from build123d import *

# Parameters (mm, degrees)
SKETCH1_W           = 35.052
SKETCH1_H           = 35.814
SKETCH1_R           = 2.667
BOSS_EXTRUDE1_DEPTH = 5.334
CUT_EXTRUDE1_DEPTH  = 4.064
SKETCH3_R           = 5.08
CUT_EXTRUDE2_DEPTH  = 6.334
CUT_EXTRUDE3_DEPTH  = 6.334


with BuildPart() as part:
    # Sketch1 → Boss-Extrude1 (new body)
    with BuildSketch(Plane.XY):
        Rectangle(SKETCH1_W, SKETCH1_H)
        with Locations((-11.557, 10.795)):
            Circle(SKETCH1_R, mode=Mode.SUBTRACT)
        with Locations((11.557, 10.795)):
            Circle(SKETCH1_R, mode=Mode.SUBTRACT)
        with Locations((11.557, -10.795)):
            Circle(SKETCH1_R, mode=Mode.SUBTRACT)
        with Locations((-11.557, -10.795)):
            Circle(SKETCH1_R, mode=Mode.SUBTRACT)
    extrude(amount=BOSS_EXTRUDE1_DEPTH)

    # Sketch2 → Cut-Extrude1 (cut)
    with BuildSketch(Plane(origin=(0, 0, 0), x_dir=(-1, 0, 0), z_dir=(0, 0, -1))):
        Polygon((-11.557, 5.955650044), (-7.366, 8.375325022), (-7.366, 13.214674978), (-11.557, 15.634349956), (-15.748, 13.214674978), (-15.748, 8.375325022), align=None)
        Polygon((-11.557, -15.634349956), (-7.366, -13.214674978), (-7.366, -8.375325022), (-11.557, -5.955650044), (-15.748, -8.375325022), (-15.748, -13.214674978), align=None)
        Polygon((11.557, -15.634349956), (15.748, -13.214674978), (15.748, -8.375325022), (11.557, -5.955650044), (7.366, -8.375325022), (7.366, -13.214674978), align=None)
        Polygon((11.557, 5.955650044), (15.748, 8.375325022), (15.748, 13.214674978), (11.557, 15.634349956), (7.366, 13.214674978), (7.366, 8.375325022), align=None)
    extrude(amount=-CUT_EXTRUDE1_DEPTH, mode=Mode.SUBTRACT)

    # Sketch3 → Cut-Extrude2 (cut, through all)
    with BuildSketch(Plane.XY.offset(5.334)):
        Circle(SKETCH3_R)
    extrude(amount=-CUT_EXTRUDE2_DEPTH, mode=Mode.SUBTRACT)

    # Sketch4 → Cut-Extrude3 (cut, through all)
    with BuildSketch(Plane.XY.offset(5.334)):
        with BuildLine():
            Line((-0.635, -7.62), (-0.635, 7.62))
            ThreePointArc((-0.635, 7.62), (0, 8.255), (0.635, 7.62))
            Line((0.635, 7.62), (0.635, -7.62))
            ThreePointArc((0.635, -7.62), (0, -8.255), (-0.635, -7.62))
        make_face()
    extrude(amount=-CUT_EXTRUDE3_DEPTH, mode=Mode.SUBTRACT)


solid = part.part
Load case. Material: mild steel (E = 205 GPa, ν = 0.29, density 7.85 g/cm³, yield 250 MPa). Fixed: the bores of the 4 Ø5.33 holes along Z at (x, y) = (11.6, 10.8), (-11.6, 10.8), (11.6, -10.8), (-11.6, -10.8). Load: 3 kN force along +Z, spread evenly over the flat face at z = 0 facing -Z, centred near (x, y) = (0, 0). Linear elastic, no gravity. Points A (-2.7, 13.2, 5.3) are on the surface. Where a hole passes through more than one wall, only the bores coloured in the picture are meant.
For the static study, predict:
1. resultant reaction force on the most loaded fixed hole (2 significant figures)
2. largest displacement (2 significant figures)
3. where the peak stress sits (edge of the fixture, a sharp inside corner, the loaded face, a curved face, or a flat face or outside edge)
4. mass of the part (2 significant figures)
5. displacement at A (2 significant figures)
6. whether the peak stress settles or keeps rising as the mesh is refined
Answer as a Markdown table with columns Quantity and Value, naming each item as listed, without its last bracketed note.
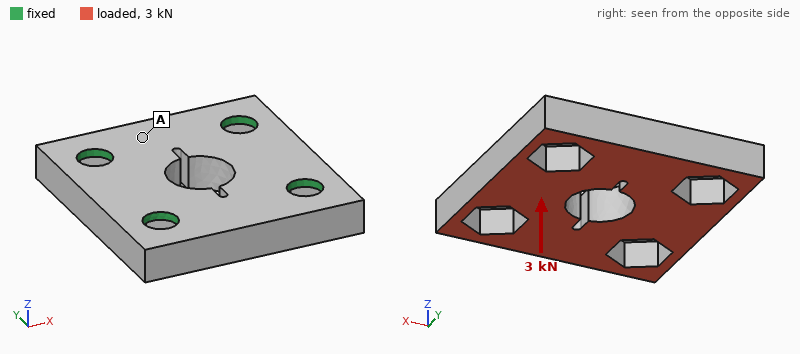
| Quantity | Value |
|---|---|
| resultant reaction force on the most loaded fixed hole | 800 N |
| largest displacement | 4.1 µm |
| where the peak stress sits | edge of the fixture |
| mass of the part | 40 g |
| displacement at A | 3.1 µm |
| whether the peak stress settles or keeps rising as the mesh is refined | keeps rising |
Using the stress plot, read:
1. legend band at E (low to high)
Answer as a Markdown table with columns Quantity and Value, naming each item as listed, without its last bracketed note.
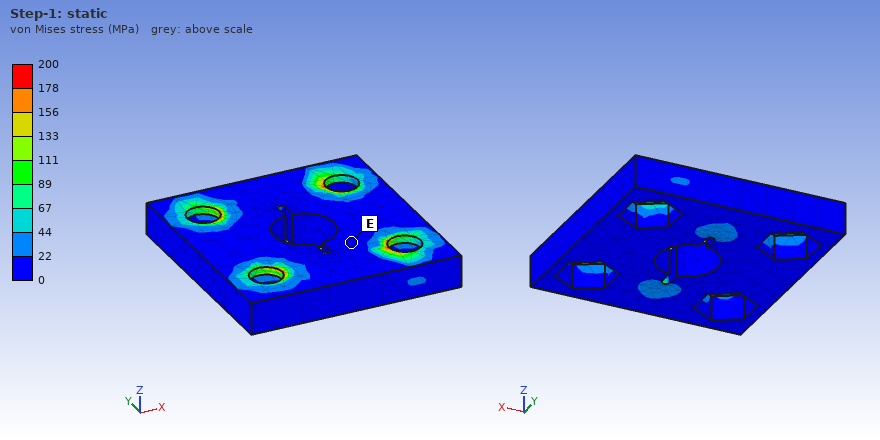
| Quantity | Value |
|---|---|
| legend band at E | 0 to 22 MPa |
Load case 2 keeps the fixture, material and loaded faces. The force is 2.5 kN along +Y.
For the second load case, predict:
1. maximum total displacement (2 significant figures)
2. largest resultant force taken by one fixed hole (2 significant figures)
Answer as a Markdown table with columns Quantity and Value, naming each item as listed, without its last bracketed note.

| Quantity | Value |
|---|---|
| maximum total displacement | 3.5 µm |
| largest resultant force taken by one fixed hole | 680 N |
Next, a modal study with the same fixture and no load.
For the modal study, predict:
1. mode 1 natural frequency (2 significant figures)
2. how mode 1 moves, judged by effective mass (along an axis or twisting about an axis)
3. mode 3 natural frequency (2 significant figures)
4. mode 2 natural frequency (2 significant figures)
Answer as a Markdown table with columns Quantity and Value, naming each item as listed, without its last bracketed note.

| Quantity | Value |
|---|---|
| mode 1 natural frequency | 25 kHz |
| how mode 1 moves, judged by effective mass | along Z |
| mode 3 natural frequency | 28 kHz |
| mode 2 natural frequency | 27 kHz |
